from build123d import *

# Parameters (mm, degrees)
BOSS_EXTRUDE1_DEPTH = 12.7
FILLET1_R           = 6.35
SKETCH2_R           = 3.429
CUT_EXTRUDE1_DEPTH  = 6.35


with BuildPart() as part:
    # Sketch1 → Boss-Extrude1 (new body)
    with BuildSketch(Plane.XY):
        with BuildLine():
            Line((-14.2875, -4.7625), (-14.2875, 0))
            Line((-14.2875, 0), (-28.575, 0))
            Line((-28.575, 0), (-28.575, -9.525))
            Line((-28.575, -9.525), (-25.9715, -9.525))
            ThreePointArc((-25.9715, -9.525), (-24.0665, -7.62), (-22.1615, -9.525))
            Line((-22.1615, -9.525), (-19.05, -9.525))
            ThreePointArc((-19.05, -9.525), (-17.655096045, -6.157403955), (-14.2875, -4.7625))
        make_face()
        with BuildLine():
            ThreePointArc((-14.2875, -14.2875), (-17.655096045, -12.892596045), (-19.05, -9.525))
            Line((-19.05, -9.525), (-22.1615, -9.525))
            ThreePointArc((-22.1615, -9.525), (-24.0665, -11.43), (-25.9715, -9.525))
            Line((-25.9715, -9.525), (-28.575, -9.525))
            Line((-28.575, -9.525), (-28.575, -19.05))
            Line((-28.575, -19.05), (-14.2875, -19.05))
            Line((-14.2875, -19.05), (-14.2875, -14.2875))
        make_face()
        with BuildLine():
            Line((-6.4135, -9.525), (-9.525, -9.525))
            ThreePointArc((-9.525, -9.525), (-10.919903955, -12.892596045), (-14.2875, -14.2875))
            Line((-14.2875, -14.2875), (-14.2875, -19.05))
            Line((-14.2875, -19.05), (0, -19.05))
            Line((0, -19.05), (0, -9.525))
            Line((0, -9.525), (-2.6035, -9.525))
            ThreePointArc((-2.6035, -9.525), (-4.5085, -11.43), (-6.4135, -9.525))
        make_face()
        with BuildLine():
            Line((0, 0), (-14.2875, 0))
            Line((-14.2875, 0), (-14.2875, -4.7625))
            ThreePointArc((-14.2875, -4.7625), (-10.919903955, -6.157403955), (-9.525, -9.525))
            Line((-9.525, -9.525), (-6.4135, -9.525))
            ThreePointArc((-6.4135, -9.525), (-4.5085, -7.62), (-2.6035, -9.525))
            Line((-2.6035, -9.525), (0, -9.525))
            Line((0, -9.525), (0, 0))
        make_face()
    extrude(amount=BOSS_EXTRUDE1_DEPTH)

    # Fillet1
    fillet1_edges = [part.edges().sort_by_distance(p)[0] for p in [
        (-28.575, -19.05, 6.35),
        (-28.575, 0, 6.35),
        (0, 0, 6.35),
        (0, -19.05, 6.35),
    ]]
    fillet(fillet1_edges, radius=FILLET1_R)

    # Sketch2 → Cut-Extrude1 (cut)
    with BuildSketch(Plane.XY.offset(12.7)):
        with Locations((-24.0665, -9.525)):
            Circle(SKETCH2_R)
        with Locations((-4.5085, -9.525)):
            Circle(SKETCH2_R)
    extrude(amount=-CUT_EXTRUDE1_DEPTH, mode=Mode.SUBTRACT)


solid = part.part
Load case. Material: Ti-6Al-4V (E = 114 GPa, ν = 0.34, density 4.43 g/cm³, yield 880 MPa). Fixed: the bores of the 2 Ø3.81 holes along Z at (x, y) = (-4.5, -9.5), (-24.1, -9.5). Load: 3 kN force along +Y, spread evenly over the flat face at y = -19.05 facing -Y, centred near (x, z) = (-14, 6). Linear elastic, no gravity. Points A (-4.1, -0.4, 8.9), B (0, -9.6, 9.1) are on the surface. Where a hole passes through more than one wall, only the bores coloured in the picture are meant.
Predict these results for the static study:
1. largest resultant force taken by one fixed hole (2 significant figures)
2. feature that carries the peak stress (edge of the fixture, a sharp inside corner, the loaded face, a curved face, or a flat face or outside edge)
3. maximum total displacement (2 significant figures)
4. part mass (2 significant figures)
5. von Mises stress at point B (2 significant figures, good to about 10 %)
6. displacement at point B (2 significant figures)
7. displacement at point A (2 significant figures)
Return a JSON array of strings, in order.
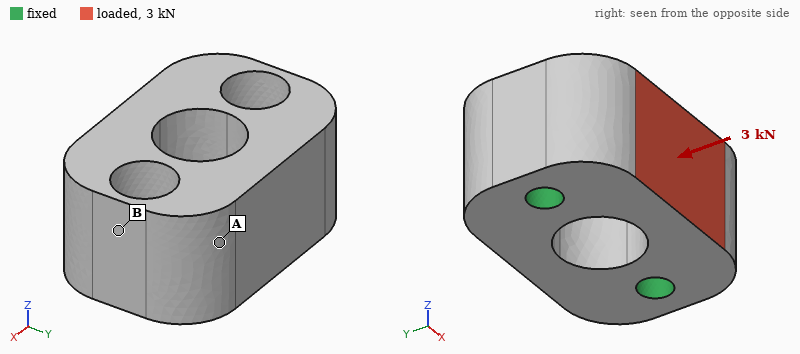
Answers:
["1.6 kN", "edge of the fixture", "9.9 µm", "22 g", "23 MPa", "2.3 µm", "3.6 µm"]
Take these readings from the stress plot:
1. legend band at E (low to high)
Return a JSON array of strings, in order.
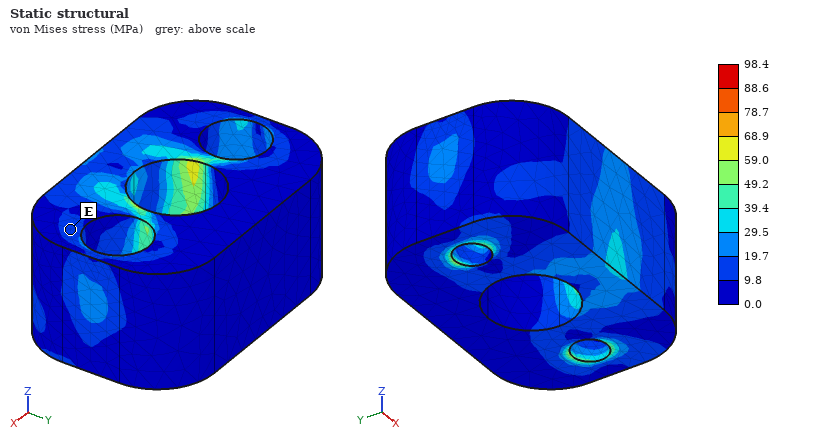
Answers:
["9.8 to 19.7 MPa"]
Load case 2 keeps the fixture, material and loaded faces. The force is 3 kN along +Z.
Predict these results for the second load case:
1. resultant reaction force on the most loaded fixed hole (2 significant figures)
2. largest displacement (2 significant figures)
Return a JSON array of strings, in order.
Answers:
["1.6 kN", "24 µm"]
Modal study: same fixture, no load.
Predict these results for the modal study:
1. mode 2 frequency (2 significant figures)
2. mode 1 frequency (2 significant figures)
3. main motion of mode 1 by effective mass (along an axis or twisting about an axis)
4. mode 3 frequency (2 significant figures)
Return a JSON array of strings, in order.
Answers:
["41 kHz", "24 kHz", "along Y", "43 kHz"]
